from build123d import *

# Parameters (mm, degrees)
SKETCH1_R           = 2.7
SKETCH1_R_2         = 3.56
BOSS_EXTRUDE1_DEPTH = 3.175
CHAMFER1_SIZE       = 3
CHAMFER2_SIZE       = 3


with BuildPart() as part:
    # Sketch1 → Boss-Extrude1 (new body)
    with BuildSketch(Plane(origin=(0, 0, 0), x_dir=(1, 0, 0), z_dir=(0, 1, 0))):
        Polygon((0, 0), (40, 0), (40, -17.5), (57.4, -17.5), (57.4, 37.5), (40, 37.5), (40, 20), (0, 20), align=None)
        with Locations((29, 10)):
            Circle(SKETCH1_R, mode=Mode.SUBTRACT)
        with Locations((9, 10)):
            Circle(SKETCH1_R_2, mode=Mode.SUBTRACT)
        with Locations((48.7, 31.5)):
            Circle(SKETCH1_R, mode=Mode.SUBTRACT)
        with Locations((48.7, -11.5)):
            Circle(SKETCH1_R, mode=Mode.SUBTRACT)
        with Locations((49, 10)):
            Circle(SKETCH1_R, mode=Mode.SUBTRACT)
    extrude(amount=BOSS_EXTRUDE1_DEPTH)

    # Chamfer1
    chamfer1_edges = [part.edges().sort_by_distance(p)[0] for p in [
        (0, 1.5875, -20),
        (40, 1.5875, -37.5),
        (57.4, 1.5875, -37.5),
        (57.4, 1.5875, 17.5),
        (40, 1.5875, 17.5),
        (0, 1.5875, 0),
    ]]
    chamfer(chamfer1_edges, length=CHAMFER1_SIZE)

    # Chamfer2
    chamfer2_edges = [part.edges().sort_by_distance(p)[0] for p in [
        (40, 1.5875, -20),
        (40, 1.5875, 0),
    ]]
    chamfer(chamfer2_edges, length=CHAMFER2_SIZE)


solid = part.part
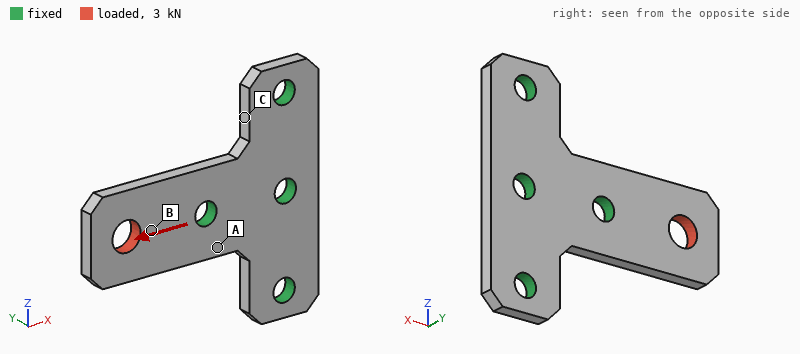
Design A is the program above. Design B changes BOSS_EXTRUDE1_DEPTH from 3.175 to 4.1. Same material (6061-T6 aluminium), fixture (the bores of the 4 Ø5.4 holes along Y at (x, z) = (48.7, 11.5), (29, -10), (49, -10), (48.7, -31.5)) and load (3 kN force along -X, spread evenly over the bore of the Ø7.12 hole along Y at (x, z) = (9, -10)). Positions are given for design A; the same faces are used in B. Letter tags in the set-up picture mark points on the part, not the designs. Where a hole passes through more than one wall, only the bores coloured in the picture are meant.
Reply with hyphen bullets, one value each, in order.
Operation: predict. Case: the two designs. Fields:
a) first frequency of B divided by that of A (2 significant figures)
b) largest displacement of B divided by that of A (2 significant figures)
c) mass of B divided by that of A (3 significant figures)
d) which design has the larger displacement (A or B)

- 1.3
- 0.78
- 1.29
- A
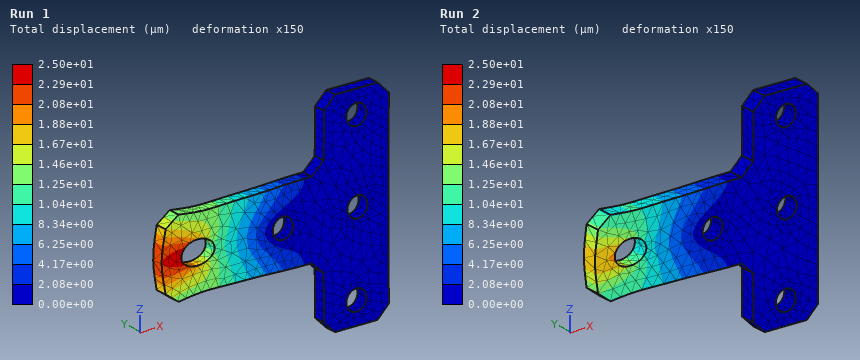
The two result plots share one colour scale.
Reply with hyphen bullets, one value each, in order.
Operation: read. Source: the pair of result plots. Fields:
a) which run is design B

- Run 2
